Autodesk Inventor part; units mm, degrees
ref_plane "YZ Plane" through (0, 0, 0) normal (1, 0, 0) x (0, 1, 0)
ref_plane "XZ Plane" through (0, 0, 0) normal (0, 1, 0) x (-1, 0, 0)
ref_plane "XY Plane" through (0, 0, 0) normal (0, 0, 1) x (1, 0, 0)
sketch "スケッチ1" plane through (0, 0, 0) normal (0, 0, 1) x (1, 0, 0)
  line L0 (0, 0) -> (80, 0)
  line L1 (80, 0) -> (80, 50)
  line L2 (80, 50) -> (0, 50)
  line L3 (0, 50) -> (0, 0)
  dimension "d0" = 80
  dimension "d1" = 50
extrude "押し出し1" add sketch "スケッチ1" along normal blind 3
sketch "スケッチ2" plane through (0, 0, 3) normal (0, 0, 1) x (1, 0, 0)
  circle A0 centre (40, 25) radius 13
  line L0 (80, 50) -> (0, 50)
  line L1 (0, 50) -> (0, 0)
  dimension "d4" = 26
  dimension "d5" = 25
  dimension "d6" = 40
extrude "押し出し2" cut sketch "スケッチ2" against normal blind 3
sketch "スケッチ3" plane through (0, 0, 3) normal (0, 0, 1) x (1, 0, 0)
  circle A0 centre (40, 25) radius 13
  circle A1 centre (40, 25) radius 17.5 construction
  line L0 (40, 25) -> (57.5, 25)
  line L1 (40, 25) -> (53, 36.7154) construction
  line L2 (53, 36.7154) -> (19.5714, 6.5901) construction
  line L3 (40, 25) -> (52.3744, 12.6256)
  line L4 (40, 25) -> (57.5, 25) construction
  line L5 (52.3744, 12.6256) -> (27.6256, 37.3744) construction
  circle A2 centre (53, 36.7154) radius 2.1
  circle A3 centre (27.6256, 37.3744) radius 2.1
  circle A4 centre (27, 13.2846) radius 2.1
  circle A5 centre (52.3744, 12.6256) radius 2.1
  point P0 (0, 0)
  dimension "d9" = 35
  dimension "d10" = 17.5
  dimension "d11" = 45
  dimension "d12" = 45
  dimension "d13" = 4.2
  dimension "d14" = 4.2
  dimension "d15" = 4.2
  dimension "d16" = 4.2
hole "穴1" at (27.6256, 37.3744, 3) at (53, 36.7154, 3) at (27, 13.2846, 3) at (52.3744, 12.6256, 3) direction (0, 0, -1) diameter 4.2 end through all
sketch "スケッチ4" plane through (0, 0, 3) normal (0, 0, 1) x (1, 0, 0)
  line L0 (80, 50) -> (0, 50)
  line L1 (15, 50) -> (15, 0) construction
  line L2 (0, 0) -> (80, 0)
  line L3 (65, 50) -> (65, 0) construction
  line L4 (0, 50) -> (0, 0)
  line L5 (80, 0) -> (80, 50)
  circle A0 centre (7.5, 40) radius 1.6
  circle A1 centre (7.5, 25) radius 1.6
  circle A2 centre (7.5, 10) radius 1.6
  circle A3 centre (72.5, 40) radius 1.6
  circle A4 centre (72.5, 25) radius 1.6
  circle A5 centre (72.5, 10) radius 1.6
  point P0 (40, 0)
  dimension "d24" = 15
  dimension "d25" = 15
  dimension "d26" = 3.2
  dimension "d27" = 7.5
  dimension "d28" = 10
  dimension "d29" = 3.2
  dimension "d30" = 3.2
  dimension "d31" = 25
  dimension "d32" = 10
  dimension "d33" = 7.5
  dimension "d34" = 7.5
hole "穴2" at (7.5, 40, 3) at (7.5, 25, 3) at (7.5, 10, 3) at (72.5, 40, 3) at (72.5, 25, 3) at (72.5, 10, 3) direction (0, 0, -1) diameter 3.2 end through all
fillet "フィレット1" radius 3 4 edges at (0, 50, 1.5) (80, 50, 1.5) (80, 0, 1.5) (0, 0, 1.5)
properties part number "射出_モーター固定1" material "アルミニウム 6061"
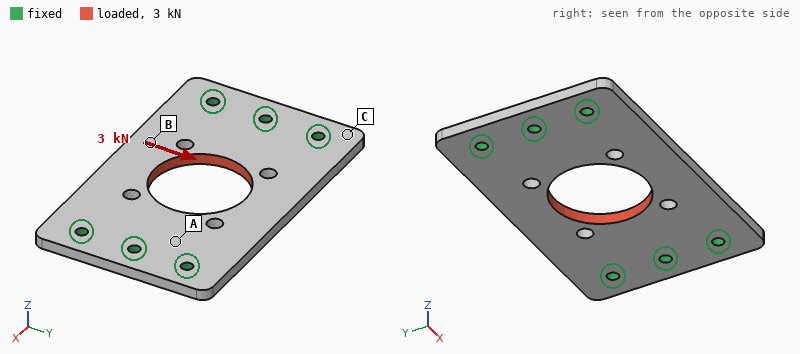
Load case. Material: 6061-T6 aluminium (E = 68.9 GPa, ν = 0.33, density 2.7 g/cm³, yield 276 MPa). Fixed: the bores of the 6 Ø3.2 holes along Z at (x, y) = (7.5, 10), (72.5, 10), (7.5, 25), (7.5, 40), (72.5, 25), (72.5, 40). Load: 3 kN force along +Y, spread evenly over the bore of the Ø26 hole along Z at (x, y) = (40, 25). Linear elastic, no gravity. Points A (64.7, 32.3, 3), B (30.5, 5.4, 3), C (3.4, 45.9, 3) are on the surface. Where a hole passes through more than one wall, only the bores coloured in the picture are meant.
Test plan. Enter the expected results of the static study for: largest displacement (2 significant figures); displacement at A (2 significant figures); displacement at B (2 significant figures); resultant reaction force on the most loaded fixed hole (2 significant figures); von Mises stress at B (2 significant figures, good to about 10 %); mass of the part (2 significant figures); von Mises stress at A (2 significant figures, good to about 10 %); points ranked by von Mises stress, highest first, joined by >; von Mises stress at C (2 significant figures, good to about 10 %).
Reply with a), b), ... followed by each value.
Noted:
a) 19 µm
b) 4.4 µm
c) 15 µm
d) 680 N
e) 18 MPa
f) 27 g
g) 26 MPa
h) A > B > C
i) 7.6 MPa
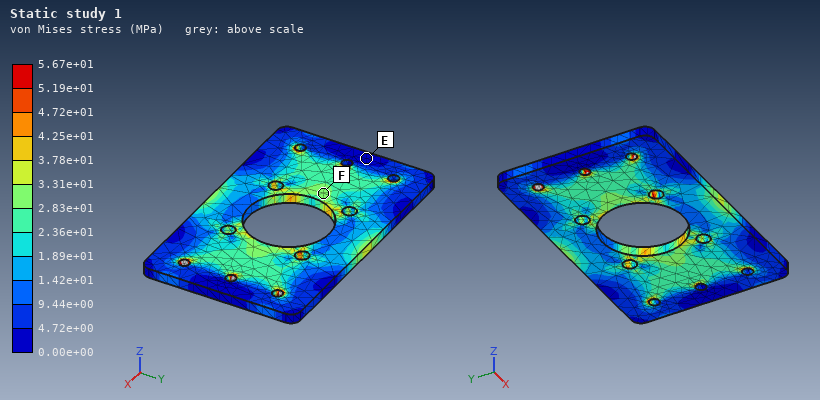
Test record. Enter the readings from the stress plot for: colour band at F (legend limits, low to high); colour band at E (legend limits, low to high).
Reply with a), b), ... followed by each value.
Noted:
a) 2.83e+01 to 3.31e+01 MPa
b) 0.00e+00 to 4.72e+00 MPa
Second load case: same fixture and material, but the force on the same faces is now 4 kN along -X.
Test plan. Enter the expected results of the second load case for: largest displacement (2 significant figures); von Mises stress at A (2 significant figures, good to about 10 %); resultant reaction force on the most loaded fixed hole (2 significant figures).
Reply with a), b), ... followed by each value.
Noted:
a) 9.0 µm
b) 14 MPa
c) 710 N
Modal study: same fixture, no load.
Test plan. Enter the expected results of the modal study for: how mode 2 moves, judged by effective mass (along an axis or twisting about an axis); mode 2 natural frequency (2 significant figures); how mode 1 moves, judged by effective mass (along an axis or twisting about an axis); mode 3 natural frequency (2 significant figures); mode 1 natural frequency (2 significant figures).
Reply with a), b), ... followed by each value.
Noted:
a) twisting about X
b) 4500 Hz
c) along Z
d) 9000 Hz
e) 4000 Hz
